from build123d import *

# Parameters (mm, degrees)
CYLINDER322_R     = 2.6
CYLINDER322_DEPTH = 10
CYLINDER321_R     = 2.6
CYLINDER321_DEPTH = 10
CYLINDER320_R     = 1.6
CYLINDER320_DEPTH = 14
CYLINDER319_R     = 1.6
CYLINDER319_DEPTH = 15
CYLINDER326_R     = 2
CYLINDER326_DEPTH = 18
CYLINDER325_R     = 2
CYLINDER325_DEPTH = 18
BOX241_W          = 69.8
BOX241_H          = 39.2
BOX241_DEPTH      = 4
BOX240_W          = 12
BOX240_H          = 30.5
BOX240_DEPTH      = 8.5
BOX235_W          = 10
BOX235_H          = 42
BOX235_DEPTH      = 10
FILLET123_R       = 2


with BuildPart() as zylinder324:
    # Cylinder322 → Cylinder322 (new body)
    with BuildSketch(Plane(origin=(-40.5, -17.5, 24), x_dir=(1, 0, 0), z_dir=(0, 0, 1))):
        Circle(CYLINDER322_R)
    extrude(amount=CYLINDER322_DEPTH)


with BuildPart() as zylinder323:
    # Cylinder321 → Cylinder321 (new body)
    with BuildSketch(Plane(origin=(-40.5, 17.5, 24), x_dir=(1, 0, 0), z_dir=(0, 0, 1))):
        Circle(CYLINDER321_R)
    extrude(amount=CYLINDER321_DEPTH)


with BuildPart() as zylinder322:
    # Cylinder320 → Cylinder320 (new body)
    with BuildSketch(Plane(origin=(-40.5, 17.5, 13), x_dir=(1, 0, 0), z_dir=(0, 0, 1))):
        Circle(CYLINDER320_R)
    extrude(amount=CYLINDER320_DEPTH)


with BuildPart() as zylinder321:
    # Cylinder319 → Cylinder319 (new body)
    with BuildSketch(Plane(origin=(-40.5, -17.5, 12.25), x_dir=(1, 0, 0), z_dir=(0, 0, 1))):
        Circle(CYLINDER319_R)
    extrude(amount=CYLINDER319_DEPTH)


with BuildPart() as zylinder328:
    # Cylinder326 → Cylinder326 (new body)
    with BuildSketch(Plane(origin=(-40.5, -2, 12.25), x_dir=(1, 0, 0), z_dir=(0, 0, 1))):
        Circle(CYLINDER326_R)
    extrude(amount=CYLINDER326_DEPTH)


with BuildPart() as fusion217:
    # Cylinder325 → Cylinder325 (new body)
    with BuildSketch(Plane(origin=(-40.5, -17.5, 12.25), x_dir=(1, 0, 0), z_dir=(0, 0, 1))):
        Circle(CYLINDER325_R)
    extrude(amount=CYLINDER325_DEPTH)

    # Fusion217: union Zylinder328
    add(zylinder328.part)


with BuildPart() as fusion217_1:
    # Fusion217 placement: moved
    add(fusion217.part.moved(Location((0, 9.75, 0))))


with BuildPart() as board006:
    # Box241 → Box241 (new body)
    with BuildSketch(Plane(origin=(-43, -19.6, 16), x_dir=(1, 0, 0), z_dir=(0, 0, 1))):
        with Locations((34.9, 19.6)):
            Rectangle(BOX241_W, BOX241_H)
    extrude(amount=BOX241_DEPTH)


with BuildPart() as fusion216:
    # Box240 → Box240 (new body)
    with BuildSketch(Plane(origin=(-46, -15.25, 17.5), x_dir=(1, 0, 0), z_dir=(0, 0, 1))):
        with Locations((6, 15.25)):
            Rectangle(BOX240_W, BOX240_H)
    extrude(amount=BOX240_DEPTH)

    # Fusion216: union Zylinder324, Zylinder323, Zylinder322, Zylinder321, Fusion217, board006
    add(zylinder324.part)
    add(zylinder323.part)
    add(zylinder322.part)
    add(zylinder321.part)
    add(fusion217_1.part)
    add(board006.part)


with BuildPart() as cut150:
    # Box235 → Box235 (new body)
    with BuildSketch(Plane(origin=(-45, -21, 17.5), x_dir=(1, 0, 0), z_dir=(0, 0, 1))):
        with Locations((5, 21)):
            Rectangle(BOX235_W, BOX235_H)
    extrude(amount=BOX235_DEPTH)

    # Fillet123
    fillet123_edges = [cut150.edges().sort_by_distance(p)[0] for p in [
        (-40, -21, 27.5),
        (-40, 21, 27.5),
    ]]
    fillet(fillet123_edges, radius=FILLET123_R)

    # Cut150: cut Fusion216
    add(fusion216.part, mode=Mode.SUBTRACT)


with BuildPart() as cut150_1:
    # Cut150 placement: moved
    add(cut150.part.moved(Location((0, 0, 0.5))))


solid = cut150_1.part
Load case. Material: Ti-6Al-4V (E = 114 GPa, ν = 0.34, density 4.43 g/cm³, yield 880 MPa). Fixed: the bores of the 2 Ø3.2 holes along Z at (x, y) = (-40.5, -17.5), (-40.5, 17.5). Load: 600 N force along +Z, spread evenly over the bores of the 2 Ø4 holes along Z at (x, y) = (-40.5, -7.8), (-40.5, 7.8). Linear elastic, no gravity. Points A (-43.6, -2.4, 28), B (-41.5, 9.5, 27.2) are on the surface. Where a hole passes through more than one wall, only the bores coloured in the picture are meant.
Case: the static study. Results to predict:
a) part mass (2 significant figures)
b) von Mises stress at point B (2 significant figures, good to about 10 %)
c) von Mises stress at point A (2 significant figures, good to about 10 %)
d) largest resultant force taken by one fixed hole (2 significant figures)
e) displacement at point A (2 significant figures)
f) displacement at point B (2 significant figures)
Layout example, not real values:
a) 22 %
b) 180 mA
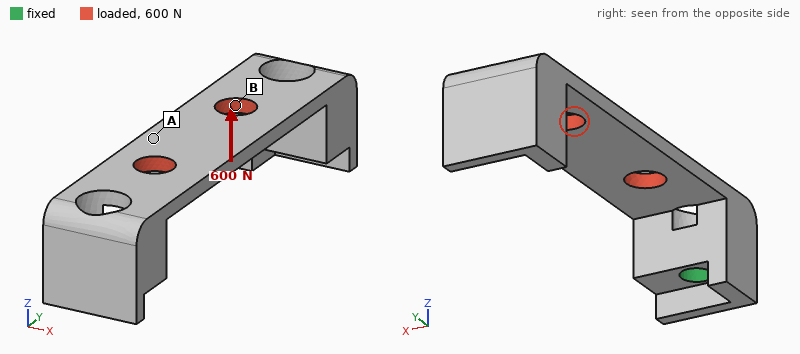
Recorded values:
a) 5.2 g
b) 75 MPa
c) 220 MPa
d) 410 N
e) 0.23 mm
f) 0.12 mm
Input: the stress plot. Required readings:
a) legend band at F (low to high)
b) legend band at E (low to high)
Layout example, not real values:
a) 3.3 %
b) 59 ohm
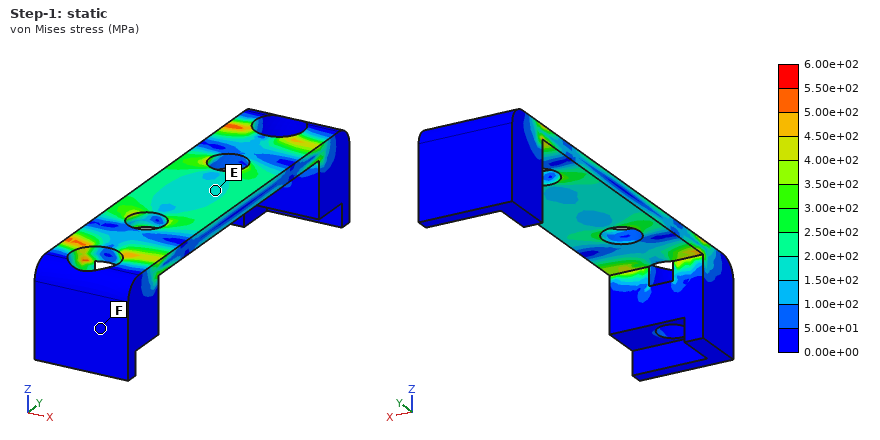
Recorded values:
a) 0.00e+00 to 5.00e+01 MPa
b) 1.50e+02 to 2.00e+02 MPa
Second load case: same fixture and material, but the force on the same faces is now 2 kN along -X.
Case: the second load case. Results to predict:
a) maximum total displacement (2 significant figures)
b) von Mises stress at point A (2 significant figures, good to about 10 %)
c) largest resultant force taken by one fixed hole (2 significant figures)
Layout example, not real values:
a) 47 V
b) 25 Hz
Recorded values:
a) 82 µm
b) 130 MPa
c) 1.0 kN
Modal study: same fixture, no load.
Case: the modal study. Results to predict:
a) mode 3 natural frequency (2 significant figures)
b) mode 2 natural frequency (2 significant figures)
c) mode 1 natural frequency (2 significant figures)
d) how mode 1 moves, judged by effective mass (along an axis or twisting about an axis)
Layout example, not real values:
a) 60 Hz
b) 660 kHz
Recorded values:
a) 18 kHz
b) 15 kHz
c) 6900 Hz
d) along Z
